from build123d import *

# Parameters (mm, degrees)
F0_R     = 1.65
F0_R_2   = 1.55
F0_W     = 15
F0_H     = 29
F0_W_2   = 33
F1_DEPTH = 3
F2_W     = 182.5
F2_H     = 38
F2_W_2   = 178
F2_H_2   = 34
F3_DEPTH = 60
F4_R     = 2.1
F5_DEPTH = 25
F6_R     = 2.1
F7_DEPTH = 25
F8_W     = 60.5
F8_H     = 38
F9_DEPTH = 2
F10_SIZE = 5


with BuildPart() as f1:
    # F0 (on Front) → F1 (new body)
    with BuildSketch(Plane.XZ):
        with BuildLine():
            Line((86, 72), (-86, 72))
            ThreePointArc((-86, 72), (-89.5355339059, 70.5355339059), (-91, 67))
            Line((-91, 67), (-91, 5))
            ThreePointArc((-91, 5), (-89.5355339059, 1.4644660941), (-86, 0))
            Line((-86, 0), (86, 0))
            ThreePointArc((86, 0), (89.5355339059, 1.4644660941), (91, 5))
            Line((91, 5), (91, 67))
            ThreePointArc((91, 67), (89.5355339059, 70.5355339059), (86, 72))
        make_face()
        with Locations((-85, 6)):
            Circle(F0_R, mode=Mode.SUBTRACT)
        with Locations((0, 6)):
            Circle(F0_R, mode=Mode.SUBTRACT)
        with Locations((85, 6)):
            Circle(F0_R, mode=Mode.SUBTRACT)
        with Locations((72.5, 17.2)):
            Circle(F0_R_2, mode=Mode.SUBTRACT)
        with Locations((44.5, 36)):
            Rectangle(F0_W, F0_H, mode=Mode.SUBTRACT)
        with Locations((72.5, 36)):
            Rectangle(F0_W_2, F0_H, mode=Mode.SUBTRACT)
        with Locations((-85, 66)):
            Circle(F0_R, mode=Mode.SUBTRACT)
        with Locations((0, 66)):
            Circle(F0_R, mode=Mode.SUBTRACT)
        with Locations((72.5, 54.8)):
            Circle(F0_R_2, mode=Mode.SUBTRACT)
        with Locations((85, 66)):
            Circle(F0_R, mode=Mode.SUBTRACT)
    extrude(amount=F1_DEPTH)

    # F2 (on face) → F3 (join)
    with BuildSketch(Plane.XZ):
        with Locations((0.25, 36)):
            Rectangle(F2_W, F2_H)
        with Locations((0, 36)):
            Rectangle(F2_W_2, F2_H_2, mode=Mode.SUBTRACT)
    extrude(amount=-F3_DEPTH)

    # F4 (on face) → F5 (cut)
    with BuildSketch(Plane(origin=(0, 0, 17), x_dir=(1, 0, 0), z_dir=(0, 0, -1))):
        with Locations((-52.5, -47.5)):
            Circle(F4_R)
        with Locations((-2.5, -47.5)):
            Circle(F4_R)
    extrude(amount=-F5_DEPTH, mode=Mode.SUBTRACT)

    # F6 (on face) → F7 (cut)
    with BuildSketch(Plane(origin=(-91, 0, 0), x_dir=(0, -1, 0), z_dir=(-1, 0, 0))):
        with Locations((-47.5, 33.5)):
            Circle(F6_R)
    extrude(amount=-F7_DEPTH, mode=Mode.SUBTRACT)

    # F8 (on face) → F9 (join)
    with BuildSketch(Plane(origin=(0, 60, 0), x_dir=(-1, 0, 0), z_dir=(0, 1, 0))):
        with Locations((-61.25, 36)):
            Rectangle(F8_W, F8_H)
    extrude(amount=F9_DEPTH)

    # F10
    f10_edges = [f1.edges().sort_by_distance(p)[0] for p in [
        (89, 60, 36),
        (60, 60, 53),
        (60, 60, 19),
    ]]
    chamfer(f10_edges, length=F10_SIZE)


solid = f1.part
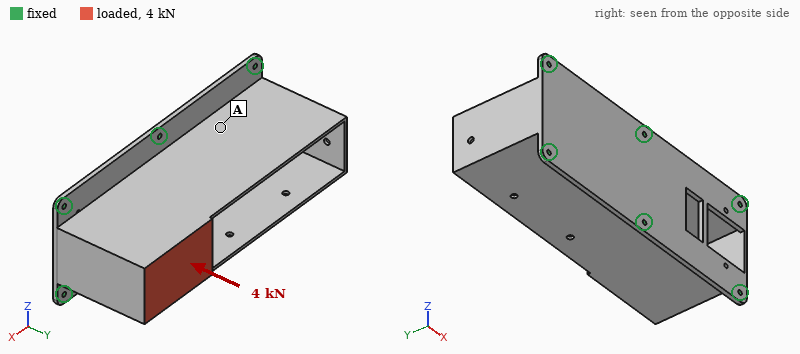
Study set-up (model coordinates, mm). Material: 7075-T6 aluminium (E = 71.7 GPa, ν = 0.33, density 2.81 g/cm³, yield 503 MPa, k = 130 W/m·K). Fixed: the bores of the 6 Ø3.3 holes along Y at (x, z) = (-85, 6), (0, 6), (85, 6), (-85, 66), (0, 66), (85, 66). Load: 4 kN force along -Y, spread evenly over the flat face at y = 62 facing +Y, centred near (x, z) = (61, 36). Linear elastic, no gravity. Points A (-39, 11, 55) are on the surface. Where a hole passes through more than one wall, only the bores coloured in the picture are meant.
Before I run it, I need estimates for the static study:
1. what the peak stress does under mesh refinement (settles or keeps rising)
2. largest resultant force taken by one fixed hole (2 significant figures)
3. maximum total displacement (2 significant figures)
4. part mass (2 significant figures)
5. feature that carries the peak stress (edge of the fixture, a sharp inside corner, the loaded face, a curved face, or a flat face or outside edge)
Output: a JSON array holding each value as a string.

["keeps rising", "1.5 kN", "0.33 mm", "260 g", "edge of the fixture"]
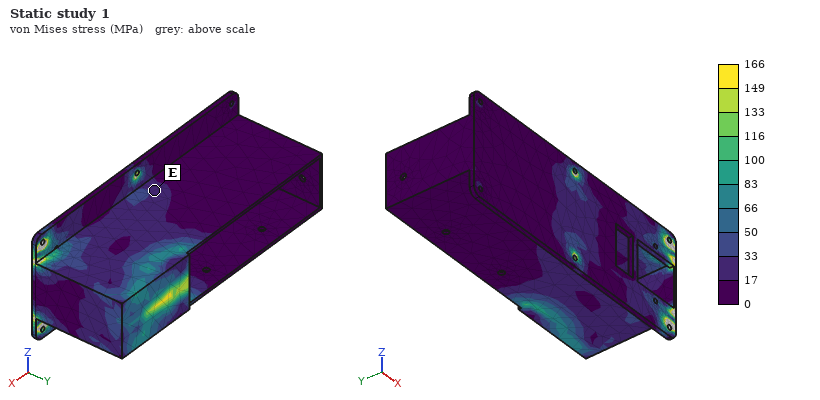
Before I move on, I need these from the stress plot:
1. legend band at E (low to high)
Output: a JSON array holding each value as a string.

["17 to 33 MPa"]
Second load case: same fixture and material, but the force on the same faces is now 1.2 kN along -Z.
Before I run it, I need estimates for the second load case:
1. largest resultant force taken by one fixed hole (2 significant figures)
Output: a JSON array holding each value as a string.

["1.5 kN"]
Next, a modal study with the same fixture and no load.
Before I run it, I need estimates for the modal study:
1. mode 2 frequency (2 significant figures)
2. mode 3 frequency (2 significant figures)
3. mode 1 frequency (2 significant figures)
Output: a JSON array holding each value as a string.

["880 Hz", "1100 Hz", "880 Hz"]
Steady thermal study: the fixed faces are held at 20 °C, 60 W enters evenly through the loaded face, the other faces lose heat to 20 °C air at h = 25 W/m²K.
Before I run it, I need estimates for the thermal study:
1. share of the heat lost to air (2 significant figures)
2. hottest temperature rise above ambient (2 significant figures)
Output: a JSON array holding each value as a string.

["52 %", "71 K"]
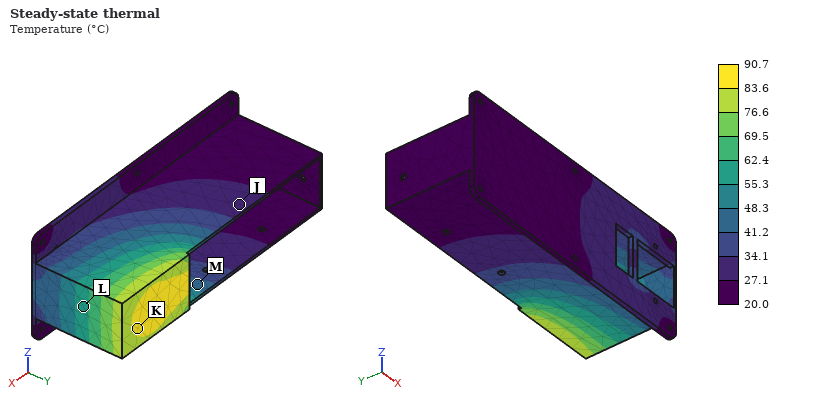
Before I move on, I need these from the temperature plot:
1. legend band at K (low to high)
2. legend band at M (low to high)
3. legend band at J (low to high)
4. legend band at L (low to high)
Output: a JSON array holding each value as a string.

["83.6 to 90.7 °C", "41.2 to 48.3 °C", "27.1 to 34.1 °C", "55.3 to 62.4 °C"]
